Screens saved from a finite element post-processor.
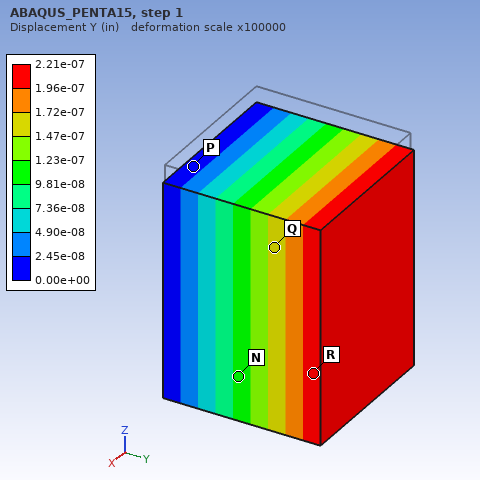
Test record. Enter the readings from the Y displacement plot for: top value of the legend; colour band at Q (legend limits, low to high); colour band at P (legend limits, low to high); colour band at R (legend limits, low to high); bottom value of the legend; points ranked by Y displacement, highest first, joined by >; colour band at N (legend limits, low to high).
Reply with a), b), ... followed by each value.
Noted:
a) 2.21e-07 in
b) 1.47e-07 to 1.72e-07 in
c) 0.00e+00 to 2.45e-08 in
d) 1.96e-07 to 2.21e-07 in
e) 0.00e+00 in
f) R > Q > N > P
g) 9.81e-08 to 1.23e-07 in
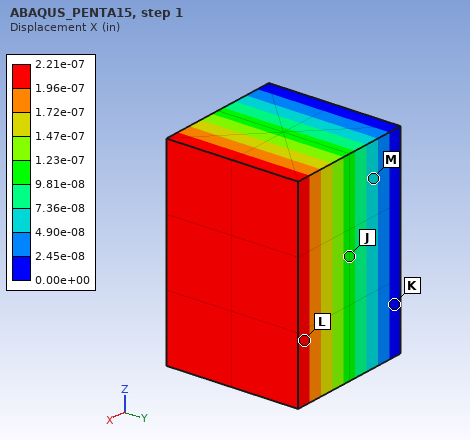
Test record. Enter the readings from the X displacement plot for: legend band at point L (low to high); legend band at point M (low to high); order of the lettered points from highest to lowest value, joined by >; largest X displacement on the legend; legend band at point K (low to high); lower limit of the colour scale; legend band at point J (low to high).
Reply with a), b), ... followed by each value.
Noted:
a) 1.96e-07 to 2.21e-07 in
b) 4.90e-08 to 7.36e-08 in
c) L > J > M > K
d) 2.21e-07 in
e) 0.00e+00 to 2.45e-08 in
f) 0.00e+00 in
g) 9.81e-08 to 1.23e-07 in
